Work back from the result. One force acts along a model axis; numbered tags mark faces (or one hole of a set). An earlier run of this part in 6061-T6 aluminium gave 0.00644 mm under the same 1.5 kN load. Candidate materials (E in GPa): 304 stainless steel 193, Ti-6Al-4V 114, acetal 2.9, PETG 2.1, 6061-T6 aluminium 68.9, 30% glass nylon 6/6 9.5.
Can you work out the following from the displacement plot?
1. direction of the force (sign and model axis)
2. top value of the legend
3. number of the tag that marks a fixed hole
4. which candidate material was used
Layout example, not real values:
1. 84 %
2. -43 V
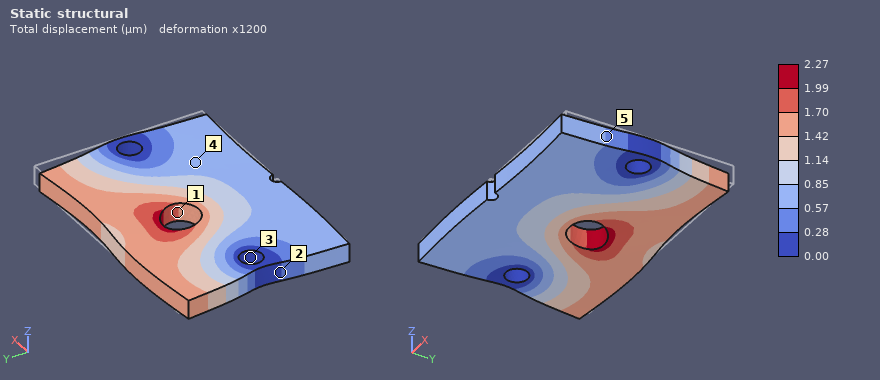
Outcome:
1. -X
2. 2.27 µm
3. 3
4. 304 stainless steel
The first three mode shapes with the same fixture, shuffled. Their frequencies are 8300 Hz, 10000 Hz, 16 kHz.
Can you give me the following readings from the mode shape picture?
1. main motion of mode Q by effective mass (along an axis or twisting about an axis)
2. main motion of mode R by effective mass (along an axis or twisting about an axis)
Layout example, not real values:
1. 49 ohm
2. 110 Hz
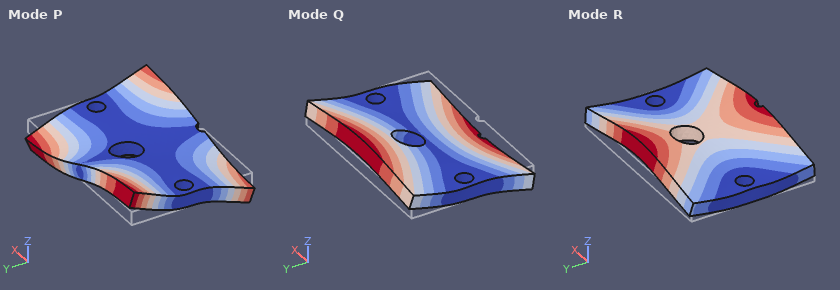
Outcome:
1. twisting about X
2. along Z
